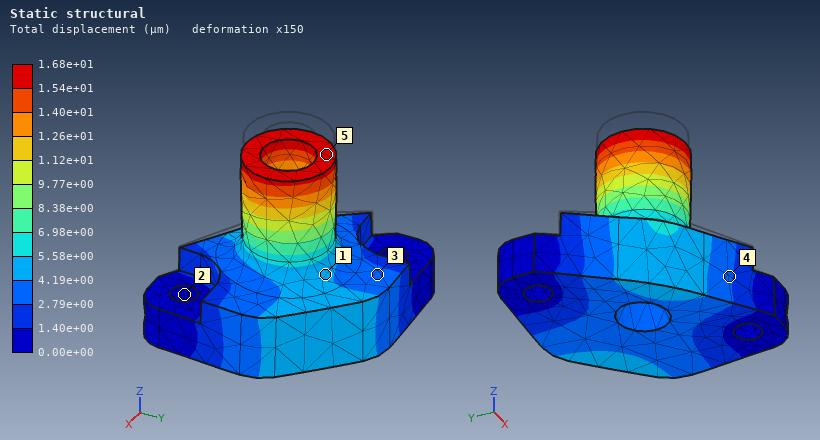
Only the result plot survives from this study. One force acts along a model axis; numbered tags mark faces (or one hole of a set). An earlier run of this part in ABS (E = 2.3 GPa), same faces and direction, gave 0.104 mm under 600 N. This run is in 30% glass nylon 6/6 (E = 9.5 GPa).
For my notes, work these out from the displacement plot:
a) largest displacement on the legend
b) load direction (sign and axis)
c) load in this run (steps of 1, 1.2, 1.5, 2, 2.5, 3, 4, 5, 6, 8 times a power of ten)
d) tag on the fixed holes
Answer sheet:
1.68e+01 µm
-Z
400 N
2
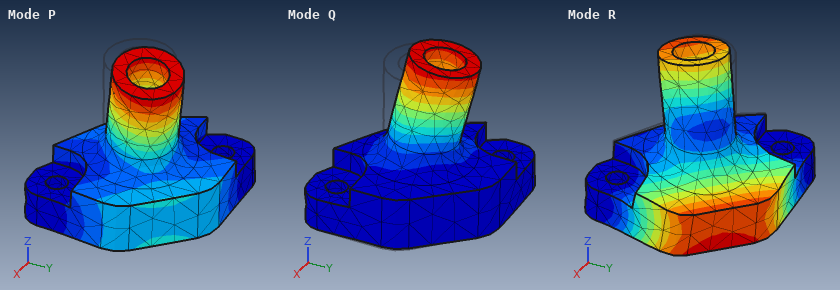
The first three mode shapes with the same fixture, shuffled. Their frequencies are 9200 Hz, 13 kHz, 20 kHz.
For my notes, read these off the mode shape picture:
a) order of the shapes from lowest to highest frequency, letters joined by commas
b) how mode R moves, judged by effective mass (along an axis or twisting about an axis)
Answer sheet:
P, Q, R
along Z
